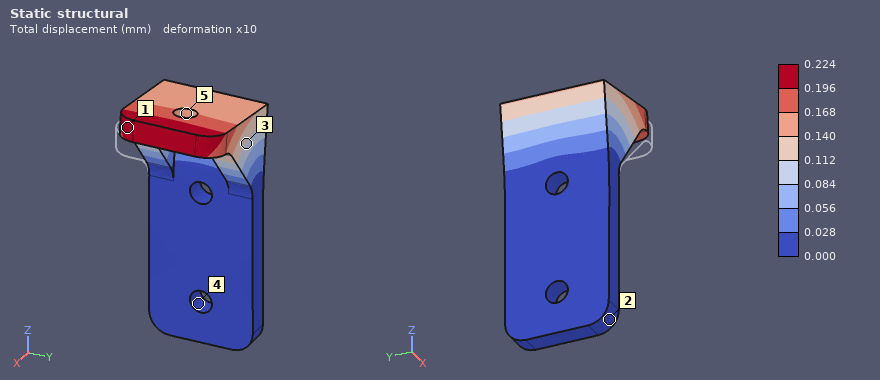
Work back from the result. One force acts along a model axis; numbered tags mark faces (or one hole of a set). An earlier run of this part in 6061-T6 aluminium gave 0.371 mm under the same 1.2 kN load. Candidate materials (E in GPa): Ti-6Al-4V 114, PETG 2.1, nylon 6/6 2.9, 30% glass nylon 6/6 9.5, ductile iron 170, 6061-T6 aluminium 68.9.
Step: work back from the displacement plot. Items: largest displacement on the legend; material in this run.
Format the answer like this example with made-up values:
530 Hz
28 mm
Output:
0.224 mm
Ti-6Al-4V
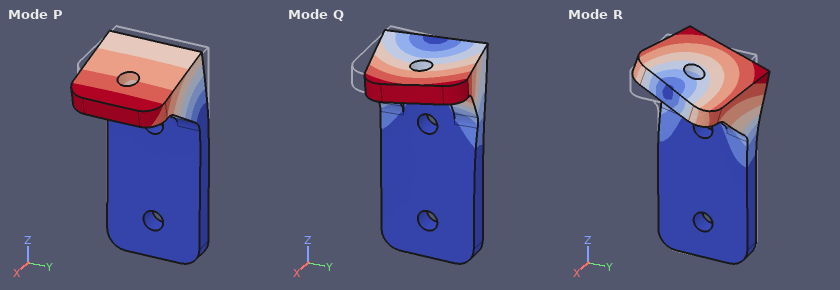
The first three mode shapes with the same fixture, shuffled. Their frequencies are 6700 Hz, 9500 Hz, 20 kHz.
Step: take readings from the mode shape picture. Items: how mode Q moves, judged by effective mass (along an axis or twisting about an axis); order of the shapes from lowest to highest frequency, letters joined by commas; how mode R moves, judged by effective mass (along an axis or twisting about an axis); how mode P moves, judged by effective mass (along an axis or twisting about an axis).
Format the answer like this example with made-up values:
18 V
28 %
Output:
along Y
P, Q, R
along Y
along X
